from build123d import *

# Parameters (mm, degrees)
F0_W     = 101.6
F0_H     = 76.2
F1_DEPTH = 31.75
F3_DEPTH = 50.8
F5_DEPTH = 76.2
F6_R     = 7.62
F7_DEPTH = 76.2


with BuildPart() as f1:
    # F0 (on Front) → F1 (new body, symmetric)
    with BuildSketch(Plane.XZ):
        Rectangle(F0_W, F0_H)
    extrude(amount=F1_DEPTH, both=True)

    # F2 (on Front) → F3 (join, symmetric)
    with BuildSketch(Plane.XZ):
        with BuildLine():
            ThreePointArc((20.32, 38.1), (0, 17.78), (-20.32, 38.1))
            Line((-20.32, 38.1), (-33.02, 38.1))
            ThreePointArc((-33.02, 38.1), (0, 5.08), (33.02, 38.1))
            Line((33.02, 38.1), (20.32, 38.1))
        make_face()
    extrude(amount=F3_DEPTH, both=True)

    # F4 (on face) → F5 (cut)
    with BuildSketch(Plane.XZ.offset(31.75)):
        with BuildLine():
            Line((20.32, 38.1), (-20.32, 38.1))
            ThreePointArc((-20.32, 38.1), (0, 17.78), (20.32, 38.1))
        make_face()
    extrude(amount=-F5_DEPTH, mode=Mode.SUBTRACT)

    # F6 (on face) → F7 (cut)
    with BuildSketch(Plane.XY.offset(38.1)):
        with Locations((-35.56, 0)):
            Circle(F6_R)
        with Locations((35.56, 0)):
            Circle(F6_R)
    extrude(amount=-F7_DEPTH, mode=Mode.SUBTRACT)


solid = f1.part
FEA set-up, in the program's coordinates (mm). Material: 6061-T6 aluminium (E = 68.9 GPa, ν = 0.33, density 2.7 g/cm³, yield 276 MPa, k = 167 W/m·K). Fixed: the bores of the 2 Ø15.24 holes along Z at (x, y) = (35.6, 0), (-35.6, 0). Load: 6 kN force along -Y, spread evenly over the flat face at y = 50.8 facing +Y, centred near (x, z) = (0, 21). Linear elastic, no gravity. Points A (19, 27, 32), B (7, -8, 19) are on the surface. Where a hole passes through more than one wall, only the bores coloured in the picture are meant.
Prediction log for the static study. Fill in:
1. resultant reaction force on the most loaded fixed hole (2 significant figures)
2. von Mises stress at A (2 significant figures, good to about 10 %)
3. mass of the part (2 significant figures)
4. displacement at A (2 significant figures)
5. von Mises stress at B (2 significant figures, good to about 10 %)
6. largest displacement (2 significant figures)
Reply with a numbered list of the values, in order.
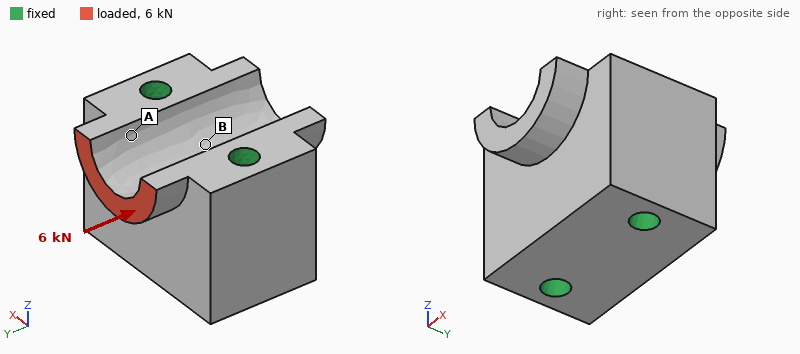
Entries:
1. 3.1 kN
2. 4.9 MPa
3. 1.3 kg
4. 2.1 µm
5. 1.1 MPa
6. 4.5 µm
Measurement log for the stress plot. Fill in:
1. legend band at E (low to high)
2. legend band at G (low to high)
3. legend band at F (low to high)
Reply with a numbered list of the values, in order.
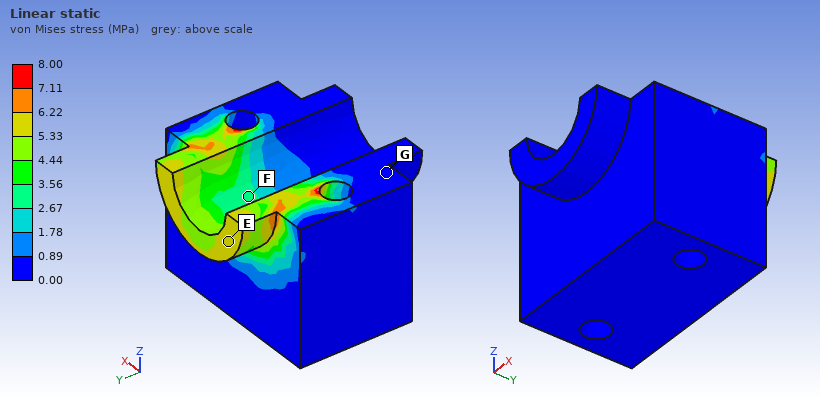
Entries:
1. 5.33 to 6.22 MPa
2. 0.00 to 0.89 MPa
3. 2.67 to 3.56 MPa
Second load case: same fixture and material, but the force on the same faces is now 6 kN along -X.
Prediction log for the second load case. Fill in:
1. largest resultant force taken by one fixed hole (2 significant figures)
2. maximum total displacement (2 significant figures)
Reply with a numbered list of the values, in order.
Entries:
1. 4.7 kN
2. 27 µm
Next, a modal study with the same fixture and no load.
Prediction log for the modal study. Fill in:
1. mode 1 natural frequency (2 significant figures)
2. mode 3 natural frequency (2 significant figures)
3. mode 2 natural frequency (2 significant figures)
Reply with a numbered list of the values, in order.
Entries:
1. 14 kHz
2. 15 kHz
3. 15 kHz
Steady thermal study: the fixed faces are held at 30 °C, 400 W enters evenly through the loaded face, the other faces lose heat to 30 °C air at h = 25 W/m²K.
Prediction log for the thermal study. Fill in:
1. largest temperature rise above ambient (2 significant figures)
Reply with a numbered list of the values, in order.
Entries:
1. 72 K
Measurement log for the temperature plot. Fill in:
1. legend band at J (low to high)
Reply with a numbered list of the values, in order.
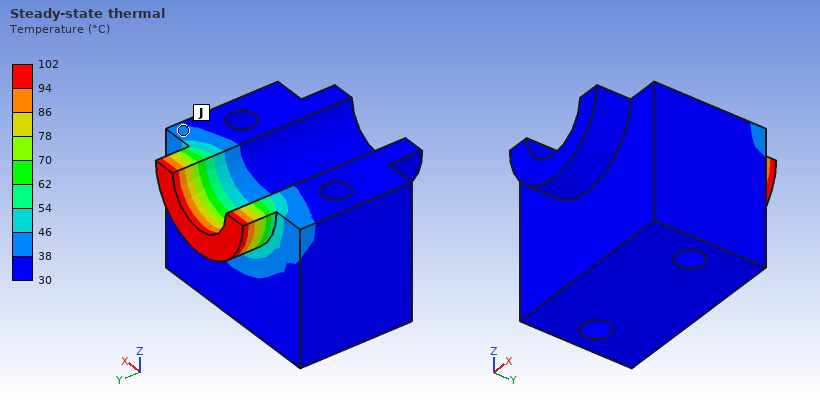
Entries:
1. 38 to 46 °C
